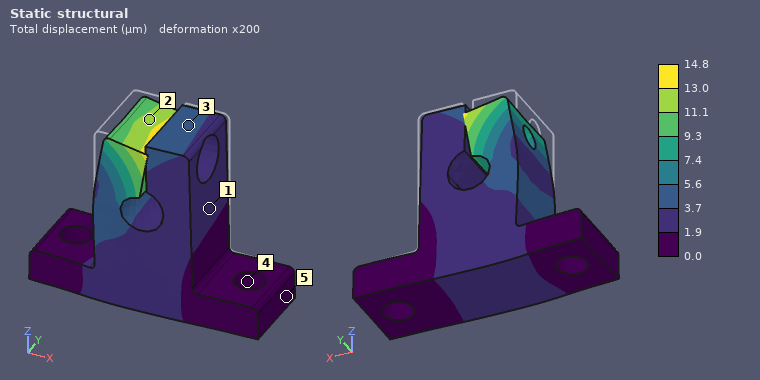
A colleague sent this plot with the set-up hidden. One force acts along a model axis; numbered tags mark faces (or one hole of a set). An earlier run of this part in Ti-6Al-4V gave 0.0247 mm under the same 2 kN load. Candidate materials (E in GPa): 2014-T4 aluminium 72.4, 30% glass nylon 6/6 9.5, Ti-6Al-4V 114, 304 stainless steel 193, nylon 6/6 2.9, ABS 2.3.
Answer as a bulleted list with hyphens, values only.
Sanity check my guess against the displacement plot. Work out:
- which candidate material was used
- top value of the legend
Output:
- 304 stainless steel
- 14.8 µm
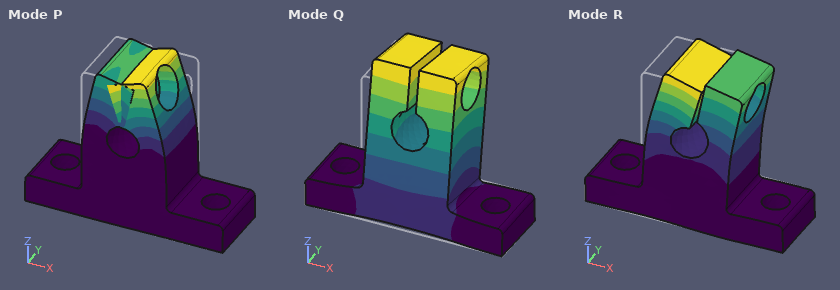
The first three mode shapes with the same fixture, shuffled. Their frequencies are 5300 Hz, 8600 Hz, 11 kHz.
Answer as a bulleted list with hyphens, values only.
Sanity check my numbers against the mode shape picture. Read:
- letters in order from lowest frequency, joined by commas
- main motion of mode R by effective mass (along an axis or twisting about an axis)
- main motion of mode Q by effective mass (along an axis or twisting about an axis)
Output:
- Q, R, P
- along X
- along Y
